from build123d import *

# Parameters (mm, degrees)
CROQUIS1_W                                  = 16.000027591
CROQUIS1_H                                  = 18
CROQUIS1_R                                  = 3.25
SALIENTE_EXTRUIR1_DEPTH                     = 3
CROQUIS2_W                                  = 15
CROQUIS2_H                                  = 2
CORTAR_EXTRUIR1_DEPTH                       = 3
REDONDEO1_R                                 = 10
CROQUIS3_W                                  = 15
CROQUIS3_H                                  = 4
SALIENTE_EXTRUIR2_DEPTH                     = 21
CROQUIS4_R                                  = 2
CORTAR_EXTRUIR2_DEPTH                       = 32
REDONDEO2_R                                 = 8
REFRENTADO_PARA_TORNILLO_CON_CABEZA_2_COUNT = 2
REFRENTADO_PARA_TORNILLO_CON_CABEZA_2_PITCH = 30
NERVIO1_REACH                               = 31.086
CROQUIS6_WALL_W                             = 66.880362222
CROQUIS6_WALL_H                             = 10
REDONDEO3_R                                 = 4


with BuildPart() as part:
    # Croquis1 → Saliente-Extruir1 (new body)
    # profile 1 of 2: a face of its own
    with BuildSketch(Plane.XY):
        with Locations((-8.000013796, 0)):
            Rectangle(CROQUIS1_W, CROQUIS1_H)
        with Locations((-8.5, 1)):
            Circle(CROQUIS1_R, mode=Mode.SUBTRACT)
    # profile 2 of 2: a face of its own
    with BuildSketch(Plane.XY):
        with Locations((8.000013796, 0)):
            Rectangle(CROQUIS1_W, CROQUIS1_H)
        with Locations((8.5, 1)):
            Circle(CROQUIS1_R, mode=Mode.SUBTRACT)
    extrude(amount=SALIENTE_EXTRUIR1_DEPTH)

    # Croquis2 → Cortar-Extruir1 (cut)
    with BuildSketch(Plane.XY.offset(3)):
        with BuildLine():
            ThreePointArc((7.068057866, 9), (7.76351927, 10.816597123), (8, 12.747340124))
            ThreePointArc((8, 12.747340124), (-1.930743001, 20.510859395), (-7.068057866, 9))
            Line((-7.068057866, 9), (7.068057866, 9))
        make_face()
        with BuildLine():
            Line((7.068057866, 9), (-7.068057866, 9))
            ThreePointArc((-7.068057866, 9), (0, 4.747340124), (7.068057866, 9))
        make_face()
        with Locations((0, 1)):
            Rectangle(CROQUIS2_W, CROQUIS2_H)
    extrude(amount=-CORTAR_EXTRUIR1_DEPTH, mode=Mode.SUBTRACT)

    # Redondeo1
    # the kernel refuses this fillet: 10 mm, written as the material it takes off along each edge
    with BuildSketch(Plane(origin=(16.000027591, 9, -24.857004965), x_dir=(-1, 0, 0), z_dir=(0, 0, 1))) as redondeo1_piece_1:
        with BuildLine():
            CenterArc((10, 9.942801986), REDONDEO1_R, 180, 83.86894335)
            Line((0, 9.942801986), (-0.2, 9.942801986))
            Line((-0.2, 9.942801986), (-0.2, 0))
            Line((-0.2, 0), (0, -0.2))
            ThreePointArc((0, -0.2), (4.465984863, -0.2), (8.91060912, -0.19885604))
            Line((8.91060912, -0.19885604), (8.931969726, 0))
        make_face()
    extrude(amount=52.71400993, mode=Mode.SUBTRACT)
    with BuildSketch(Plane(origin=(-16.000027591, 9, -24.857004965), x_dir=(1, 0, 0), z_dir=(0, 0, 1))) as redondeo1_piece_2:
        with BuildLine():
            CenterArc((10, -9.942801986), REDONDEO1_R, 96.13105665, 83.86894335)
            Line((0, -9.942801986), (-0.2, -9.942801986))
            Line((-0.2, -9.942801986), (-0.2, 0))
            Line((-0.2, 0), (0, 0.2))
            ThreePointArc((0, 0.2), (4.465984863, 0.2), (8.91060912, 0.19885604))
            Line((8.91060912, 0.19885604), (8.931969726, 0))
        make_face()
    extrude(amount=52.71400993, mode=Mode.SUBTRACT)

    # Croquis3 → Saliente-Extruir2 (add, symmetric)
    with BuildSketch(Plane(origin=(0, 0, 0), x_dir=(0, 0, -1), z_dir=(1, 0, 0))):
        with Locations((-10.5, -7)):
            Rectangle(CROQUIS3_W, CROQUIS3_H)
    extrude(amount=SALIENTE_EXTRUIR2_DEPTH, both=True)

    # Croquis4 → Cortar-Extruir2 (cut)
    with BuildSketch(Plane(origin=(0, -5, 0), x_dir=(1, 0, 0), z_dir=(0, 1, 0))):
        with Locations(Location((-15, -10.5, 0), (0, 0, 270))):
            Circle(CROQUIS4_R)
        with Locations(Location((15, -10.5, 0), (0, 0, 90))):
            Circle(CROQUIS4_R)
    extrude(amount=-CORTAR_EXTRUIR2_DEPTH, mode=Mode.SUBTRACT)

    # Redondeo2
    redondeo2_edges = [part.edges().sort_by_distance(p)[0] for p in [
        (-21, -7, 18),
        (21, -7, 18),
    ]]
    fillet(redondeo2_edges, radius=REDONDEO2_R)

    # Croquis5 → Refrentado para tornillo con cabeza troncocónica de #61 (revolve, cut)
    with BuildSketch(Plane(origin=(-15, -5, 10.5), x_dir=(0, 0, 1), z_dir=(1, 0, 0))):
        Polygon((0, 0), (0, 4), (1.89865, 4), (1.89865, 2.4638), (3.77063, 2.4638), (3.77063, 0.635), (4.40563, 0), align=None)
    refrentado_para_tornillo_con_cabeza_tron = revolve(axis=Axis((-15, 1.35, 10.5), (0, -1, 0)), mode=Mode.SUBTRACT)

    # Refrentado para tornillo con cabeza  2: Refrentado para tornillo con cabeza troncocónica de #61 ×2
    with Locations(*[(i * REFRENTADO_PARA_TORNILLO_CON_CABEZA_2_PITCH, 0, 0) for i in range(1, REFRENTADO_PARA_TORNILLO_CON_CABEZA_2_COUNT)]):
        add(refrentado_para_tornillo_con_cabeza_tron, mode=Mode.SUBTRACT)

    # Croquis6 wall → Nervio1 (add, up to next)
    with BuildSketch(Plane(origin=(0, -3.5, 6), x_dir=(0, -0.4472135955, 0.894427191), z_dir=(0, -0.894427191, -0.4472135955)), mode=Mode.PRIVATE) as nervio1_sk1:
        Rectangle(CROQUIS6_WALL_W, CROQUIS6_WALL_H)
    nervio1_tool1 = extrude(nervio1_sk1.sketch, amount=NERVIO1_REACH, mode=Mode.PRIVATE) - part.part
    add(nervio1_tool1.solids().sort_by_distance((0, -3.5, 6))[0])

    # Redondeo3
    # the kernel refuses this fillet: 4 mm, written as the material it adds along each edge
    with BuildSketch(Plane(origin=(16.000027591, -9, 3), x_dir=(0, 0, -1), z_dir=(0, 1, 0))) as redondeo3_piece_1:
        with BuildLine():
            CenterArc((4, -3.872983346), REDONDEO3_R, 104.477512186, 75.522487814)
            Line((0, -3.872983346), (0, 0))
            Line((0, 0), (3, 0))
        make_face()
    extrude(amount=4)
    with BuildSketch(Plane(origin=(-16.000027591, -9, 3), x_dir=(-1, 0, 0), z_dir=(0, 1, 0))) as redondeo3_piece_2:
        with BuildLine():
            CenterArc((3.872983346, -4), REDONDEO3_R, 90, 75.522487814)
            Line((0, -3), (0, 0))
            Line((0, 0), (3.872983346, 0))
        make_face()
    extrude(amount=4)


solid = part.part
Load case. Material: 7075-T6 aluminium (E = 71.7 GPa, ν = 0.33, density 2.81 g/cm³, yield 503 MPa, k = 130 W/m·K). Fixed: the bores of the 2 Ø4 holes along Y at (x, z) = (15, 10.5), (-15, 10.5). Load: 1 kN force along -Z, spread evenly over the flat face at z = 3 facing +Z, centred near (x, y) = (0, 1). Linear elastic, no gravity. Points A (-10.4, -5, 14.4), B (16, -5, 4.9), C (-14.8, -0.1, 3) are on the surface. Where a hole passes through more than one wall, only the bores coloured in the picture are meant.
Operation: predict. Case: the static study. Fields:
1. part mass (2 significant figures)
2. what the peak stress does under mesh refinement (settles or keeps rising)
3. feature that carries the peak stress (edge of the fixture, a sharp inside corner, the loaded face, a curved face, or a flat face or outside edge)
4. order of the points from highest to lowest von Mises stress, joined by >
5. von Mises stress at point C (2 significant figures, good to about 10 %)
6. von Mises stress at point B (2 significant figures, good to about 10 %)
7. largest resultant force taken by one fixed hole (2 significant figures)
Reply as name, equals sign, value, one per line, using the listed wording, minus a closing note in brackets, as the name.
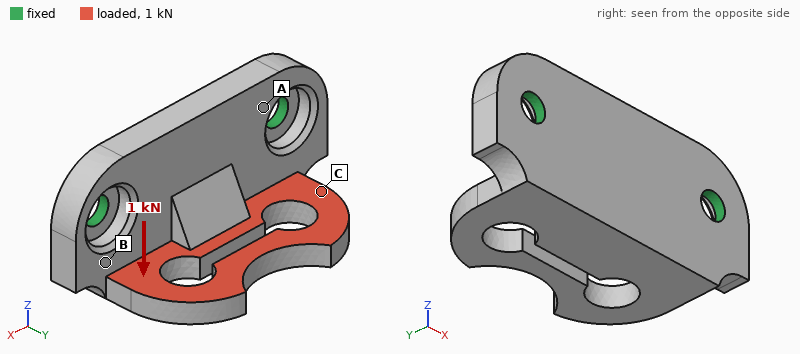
part mass = 9.7 g
what the peak stress does under mesh refinement = keeps rising
feature that carries the peak stress = edge of the fixture
order of the points from highest to lowest von Mises stress, joined by > = C > B > A
von Mises stress at point C = 190 MPa
von Mises stress at point B = 110 MPa
largest resultant force taken by one fixed hole = 500 N
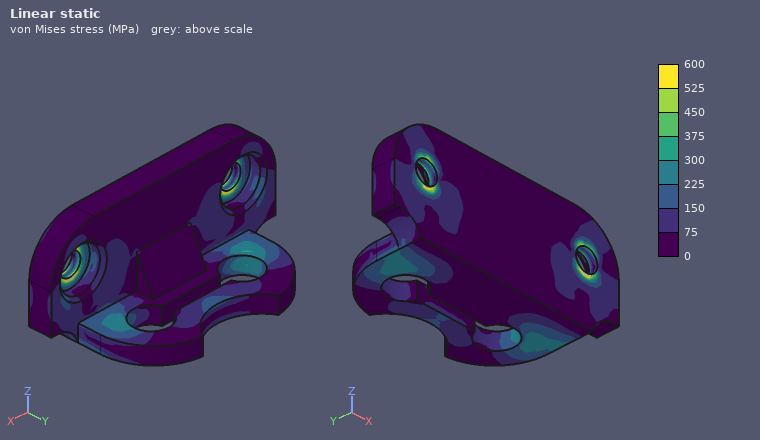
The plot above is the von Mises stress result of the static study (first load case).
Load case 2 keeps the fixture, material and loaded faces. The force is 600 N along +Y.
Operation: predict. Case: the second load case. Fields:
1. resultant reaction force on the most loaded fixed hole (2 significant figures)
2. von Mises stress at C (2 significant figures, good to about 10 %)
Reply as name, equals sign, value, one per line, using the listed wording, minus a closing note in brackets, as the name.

resultant reaction force on the most loaded fixed hole = 320 N
von Mises stress at C = 36 MPa
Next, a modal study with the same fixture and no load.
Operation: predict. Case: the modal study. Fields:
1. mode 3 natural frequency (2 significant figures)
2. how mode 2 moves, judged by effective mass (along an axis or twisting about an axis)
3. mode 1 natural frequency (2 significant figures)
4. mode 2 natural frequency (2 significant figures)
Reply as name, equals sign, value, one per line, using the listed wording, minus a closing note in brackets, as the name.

mode 3 natural frequency = 12 kHz
how mode 2 moves, judged by effective mass = along Y
mode 1 natural frequency = 5400 Hz
mode 2 natural frequency = 11 kHz
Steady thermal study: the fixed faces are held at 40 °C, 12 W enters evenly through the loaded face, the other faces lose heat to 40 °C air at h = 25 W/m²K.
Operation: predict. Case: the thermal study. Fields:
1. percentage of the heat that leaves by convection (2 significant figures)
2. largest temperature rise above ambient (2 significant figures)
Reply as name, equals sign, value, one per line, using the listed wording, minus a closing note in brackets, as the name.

percentage of the heat that leaves by convection = 5.1 %
largest temperature rise above ambient = 38 K
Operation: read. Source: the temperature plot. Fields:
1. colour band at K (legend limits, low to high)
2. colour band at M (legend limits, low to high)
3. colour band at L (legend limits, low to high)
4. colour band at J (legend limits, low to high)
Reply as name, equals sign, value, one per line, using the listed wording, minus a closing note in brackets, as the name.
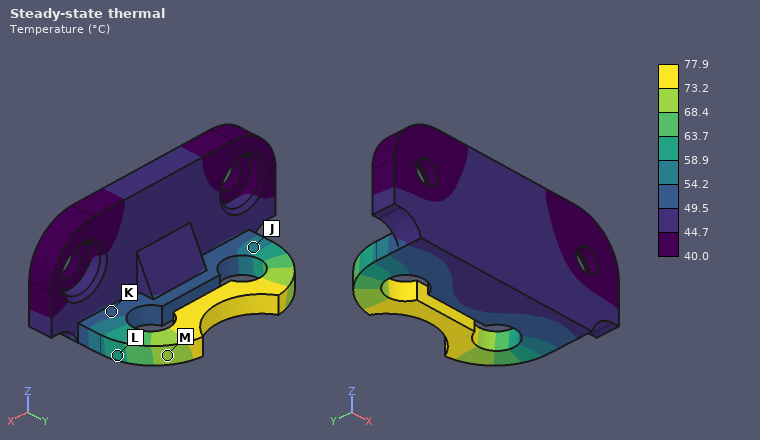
colour band at K = 49.5 to 54.2 °C
colour band at M = 68.4 to 73.2 °C
colour band at L = 58.9 to 63.7 °C
colour band at J = 54.2 to 58.9 °C
